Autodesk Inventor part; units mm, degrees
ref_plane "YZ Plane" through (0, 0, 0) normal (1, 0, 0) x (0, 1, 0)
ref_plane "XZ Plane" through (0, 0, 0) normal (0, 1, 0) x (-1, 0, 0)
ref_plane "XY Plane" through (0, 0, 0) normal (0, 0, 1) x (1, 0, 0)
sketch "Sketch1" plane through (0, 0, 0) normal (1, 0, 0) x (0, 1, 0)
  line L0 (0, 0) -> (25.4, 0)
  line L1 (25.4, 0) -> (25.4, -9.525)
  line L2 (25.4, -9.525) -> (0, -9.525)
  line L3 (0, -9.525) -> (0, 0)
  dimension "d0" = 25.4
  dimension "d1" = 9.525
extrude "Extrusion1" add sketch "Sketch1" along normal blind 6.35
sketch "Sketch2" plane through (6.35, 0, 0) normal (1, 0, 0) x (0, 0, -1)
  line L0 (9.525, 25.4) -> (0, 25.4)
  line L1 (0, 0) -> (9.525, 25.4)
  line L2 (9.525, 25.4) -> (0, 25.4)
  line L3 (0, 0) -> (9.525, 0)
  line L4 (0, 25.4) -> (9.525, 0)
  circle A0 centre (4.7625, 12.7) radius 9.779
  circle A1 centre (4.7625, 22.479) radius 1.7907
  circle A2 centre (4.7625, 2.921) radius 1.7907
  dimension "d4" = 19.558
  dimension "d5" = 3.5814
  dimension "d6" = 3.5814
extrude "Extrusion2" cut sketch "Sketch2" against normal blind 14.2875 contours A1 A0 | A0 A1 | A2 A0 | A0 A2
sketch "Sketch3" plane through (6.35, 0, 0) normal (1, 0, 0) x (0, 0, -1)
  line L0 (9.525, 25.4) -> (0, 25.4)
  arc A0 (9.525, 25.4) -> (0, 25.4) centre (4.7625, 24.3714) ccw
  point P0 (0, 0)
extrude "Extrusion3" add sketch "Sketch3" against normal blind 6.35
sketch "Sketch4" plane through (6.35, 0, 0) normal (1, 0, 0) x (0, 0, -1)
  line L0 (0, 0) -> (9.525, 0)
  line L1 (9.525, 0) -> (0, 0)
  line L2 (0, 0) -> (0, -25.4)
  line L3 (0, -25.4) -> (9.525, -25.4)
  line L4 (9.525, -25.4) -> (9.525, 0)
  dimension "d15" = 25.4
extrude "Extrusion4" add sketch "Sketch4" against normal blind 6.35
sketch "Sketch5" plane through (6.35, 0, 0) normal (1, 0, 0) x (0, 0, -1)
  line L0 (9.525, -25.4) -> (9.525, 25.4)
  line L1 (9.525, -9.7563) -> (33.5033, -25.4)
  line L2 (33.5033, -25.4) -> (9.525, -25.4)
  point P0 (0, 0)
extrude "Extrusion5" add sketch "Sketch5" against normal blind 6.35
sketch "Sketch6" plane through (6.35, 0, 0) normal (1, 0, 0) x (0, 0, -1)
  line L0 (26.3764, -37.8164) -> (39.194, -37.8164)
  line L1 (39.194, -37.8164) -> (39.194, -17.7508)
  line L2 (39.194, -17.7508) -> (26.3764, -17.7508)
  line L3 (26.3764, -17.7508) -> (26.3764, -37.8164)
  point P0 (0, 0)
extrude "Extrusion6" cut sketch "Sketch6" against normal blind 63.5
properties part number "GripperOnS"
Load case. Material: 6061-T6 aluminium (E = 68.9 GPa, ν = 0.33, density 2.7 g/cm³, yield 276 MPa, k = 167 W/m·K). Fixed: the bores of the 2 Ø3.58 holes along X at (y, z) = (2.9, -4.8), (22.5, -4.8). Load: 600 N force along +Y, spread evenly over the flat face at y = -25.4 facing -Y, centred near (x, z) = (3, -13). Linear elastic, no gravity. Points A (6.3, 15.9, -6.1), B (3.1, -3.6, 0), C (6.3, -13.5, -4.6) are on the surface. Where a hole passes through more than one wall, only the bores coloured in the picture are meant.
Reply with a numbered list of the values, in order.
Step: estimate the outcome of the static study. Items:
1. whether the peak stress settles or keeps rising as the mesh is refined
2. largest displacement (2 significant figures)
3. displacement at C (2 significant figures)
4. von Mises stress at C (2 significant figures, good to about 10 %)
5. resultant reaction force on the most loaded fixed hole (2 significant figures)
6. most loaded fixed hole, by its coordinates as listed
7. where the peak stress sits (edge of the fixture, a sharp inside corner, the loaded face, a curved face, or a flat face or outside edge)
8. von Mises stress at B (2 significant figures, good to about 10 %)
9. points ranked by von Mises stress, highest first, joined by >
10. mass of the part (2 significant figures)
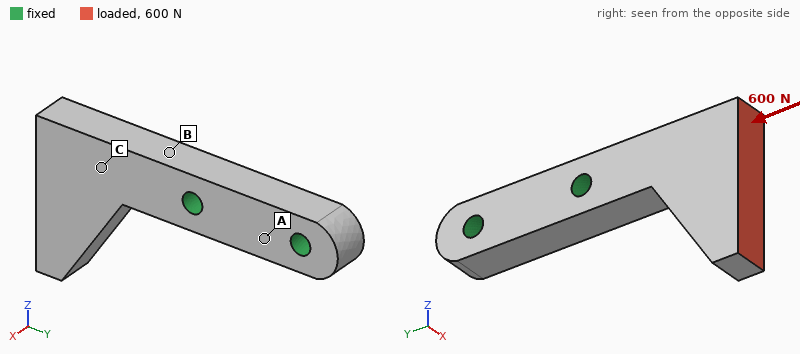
1. keeps rising
2. 100 µm
3. 27 µm
4. 16 MPa
5. 580 N
6. (2.9, -4.8)
7. edge of the fixture
8. 44 MPa
9. B > C > A
10. 11 g
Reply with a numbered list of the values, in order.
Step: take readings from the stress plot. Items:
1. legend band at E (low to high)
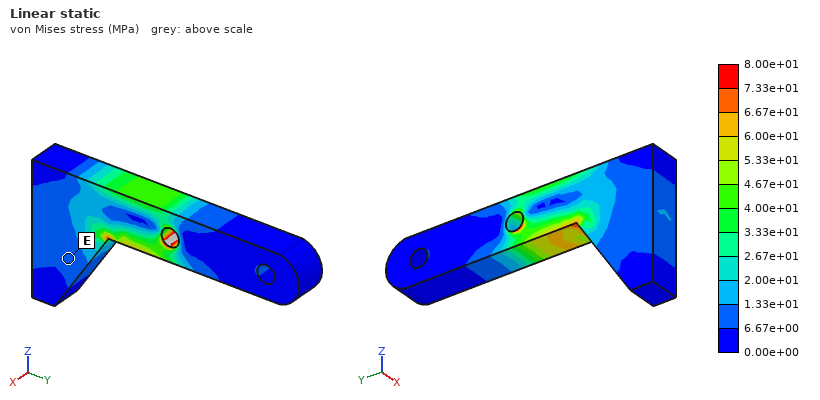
1. 6.67e+00 to 1.33e+01 MPa
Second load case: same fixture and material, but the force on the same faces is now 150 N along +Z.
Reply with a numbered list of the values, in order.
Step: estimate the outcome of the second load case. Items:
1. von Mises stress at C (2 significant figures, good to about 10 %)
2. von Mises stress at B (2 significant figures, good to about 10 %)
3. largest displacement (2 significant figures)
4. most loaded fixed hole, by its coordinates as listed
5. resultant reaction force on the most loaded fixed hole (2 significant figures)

1. 9.5 MPa
2. 34 MPa
3. 63 µm
4. (2.9, -4.8)
5. 230 N
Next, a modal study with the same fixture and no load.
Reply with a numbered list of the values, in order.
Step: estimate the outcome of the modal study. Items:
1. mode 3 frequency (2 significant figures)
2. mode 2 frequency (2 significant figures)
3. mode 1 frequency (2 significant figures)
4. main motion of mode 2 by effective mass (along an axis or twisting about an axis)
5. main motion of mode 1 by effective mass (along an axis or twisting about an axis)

1. 9000 Hz
2. 4700 Hz
3. 3700 Hz
4. along Z
5. along X
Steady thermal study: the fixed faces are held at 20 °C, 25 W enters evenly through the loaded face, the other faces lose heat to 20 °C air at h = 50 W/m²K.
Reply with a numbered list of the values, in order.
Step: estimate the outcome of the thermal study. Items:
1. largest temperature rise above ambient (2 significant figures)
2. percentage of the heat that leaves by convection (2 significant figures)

1. 58 K
2. 9.1 %
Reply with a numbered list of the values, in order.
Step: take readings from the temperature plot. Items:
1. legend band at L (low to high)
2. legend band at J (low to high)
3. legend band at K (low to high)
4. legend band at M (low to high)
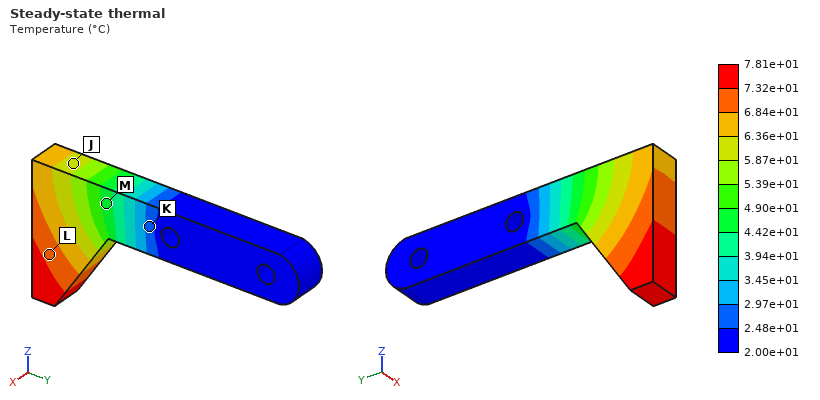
1. 6.84e+01 to 7.32e+01 °C
2. 5.87e+01 to 6.36e+01 °C
3. 2.48e+01 to 2.97e+01 °C
4. 4.42e+01 to 4.90e+01 °C
